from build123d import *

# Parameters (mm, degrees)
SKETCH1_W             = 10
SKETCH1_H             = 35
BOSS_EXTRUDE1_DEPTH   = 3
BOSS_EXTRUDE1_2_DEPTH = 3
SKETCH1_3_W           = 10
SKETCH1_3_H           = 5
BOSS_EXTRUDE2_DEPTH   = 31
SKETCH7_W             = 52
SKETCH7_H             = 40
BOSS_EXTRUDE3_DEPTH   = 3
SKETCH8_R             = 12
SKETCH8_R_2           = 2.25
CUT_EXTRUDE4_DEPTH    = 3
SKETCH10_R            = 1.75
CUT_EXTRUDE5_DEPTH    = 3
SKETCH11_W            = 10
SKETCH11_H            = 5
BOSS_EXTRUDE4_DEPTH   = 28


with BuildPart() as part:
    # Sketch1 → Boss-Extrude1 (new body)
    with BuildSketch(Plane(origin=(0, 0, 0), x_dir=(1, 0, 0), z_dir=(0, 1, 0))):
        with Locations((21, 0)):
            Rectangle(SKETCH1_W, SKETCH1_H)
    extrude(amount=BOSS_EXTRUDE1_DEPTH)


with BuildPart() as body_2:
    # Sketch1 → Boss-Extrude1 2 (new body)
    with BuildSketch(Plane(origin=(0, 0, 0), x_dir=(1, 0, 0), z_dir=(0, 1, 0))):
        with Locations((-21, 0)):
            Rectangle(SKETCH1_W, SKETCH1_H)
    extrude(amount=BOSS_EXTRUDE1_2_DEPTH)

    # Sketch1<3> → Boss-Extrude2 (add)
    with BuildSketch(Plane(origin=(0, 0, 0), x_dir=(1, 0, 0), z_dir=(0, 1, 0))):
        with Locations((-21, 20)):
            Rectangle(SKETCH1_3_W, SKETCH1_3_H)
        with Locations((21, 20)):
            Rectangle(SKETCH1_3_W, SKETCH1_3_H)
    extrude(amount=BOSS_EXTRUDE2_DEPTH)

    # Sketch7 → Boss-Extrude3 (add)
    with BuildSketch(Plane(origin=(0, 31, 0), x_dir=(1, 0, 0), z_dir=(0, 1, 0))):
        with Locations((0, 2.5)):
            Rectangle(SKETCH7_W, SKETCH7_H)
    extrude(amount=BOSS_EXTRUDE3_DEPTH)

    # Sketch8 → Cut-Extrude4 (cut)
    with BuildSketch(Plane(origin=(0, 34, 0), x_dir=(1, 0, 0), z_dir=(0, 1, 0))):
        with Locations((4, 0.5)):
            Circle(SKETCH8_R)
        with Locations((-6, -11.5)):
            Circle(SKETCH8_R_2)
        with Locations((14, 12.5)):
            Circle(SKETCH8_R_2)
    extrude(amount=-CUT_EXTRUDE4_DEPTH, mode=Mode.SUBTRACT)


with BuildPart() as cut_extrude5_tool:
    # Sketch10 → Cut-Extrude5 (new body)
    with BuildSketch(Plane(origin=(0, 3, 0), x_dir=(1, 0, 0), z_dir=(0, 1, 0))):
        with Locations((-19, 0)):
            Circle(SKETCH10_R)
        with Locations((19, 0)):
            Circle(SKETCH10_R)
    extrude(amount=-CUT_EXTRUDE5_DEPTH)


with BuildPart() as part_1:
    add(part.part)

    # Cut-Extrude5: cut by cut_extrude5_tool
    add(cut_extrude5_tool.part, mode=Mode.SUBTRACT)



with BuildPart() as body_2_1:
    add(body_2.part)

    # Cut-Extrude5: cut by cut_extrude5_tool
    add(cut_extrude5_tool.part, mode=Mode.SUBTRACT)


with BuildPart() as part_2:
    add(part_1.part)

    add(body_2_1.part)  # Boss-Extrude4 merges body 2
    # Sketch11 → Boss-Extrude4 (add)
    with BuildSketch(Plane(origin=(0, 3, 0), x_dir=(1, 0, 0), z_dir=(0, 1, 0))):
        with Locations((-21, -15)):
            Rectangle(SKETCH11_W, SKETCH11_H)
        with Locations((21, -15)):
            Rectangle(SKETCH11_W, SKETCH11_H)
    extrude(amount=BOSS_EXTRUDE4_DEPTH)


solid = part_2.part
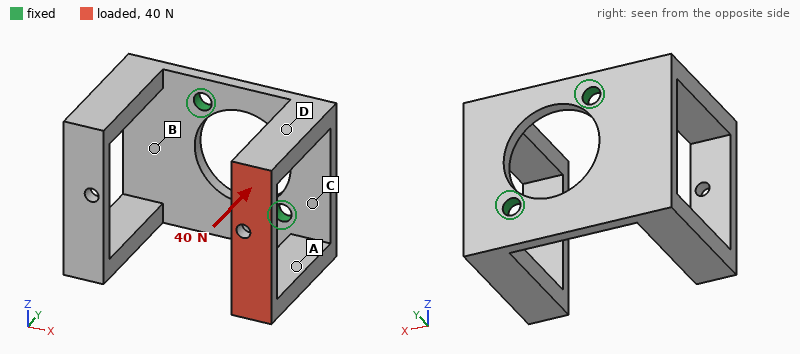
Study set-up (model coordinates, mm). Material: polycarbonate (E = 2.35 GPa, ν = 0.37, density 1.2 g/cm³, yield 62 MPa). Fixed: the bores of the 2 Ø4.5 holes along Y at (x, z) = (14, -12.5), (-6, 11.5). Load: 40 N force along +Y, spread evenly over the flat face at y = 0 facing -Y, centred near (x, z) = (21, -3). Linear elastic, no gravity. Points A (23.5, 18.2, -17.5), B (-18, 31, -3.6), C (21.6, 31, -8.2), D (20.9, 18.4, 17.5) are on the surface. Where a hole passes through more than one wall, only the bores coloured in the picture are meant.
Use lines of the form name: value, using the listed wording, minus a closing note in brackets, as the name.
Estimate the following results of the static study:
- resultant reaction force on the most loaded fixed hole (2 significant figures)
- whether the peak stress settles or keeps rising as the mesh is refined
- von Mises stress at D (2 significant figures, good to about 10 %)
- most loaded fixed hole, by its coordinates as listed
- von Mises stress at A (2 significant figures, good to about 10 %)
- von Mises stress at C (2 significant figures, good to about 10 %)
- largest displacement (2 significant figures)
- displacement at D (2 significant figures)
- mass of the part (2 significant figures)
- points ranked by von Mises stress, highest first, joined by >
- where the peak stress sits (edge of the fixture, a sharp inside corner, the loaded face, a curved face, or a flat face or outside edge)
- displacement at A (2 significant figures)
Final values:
resultant reaction force on the most loaded fixed hole: 31 N
whether the peak stress settles or keeps rising as the mesh is refined: keeps rising
von Mises stress at D: 2.0 MPa
most loaded fixed hole, by its coordinates as listed: (14, -12.5)
von Mises stress at A: 3.7 MPa
von Mises stress at C: 5.6 MPa
largest displacement: 0.86 mm
displacement at D: 0.60 mm
mass of the part: 15 g
points ranked by von Mises stress, highest first, joined by >: C > A > D > B
where the peak stress sits: edge of the fixture
displacement at A: 0.20 mm
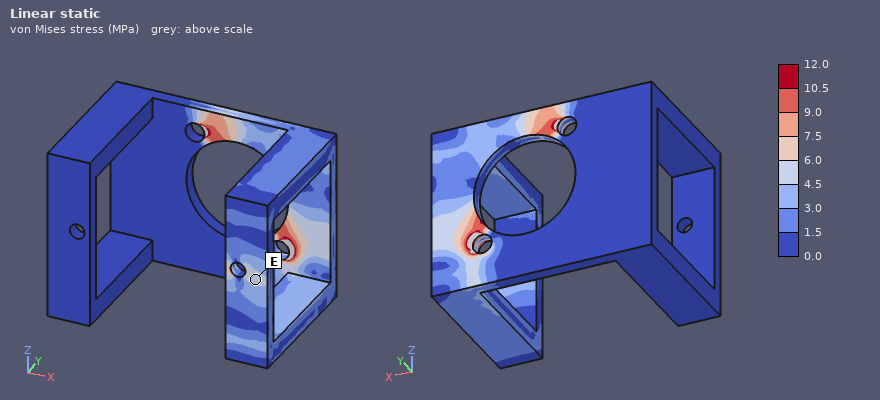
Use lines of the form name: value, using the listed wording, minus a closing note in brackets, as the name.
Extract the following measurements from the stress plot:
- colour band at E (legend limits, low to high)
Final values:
colour band at E: 4.5 to 6.0 MPa
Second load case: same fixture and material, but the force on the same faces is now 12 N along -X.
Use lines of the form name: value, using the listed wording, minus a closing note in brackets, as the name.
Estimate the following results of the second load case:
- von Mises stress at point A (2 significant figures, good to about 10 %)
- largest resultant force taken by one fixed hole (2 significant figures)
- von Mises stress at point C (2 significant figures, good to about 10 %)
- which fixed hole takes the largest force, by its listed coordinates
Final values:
von Mises stress at point A: 1.8 MPa
largest resultant force taken by one fixed hole: 8.3 N
von Mises stress at point C: 3.2 MPa
which fixed hole takes the largest force, by its listed coordinates: (14, -12.5)
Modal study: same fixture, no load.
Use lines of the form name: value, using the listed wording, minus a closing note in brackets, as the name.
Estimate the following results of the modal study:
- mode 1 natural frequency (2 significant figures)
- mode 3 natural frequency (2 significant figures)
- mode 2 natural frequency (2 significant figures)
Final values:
mode 1 natural frequency: 250 Hz
mode 3 natural frequency: 410 Hz
mode 2 natural frequency: 380 Hz
